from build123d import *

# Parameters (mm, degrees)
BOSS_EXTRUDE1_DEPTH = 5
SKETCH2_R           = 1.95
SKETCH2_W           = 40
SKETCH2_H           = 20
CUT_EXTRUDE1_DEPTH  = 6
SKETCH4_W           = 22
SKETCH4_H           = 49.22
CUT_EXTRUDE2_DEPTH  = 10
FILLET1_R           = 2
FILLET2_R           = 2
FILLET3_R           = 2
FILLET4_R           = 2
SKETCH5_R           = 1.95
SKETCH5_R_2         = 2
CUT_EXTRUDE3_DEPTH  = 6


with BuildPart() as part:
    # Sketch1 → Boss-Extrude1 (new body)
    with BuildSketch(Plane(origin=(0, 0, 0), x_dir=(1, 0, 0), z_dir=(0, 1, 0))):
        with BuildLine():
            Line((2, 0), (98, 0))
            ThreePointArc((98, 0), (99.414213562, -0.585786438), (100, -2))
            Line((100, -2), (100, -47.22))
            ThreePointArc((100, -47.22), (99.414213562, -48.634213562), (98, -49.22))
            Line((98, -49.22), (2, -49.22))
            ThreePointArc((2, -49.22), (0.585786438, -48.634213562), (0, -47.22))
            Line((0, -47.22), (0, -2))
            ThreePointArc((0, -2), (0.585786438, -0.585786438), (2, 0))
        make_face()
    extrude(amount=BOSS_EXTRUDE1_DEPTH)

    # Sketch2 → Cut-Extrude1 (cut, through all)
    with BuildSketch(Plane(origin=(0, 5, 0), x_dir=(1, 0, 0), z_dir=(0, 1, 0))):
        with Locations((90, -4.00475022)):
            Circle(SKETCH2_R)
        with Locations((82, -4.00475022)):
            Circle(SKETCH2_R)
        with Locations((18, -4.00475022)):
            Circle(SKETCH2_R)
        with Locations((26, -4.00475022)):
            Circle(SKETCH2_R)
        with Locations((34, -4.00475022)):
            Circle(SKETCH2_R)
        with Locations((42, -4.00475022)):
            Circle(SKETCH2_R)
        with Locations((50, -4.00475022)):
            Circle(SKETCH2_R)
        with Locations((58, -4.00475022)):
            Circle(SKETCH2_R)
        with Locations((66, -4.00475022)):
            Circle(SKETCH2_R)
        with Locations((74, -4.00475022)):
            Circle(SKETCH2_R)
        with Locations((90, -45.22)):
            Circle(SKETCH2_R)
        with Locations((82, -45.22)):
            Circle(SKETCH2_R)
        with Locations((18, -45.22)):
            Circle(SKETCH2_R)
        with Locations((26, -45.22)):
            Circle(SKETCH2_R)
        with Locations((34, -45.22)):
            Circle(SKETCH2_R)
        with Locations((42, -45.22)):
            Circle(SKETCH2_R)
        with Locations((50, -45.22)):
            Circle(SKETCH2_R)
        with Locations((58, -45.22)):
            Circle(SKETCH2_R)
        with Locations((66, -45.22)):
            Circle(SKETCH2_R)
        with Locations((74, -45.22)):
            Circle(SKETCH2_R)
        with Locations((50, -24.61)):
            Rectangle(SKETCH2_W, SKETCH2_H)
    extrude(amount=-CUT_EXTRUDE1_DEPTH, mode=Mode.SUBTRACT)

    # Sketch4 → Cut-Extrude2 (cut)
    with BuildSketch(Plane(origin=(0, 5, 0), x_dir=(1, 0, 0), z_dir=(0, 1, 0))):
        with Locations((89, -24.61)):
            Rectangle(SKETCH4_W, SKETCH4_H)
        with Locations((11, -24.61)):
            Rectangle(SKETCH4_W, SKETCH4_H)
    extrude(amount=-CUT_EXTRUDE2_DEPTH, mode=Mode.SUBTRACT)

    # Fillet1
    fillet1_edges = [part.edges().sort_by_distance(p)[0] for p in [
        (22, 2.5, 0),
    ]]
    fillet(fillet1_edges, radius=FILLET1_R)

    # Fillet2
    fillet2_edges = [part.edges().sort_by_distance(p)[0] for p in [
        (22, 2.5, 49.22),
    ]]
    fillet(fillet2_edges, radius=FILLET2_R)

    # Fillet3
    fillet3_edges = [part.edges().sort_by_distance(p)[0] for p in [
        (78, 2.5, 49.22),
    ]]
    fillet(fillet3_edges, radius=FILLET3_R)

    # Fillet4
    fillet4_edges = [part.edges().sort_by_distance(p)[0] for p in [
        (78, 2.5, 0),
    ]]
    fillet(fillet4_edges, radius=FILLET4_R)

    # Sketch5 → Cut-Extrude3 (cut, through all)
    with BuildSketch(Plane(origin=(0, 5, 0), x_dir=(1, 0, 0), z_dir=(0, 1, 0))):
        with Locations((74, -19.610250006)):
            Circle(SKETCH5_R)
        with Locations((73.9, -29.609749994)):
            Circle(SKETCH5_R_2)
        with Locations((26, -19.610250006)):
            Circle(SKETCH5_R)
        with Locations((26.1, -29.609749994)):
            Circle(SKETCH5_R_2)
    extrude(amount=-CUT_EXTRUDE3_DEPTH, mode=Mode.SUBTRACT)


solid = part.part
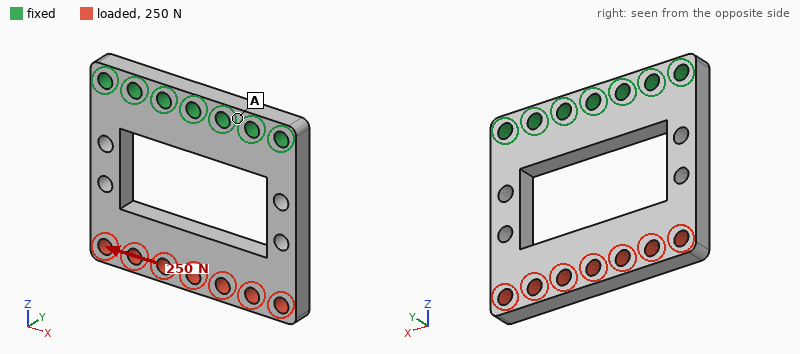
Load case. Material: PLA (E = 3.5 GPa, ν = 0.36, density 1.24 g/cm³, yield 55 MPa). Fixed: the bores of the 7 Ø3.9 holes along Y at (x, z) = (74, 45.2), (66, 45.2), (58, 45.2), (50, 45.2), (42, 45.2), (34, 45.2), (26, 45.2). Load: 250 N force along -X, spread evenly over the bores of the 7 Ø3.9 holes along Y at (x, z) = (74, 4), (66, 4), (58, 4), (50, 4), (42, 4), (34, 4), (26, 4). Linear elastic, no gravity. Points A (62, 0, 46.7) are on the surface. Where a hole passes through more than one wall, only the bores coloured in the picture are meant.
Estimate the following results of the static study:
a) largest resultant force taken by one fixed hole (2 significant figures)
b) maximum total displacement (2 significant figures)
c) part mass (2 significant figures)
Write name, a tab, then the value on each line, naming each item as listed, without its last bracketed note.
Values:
largest resultant force taken by one fixed hole	280 N
maximum total displacement	0.61 mm
part mass	11 g
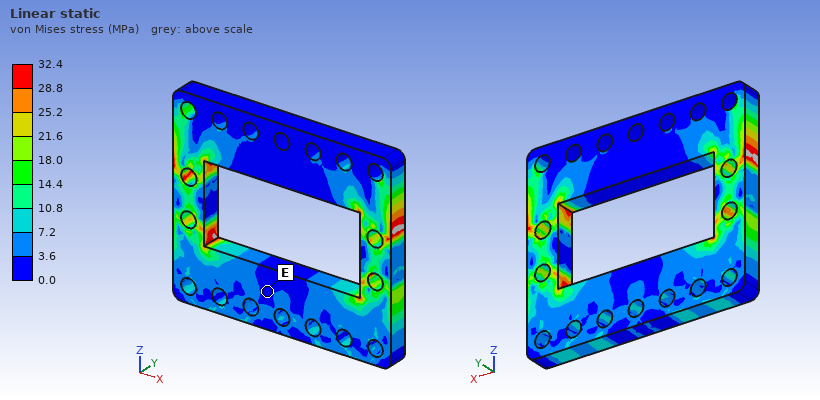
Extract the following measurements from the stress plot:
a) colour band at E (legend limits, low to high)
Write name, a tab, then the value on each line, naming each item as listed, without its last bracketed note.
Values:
colour band at E	0.0 to 3.6 MPa
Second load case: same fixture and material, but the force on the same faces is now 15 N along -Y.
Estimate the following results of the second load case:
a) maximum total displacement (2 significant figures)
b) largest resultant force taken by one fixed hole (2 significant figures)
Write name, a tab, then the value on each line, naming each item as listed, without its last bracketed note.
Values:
maximum total displacement	0.69 mm
largest resultant force taken by one fixed hole	5.9 N
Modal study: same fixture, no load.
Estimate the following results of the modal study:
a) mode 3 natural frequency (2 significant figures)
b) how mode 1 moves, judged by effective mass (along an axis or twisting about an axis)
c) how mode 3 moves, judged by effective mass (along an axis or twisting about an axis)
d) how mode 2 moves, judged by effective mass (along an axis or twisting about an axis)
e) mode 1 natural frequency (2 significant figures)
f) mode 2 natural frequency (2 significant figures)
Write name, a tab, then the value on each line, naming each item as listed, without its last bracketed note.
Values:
mode 3 natural frequency	1500 Hz
how mode 1 moves, judged by effective mass	along Y
how mode 3 moves, judged by effective mass	along X
how mode 2 moves, judged by effective mass	twisting about Z
mode 1 natural frequency	420 Hz
mode 2 natural frequency	1000 Hz
